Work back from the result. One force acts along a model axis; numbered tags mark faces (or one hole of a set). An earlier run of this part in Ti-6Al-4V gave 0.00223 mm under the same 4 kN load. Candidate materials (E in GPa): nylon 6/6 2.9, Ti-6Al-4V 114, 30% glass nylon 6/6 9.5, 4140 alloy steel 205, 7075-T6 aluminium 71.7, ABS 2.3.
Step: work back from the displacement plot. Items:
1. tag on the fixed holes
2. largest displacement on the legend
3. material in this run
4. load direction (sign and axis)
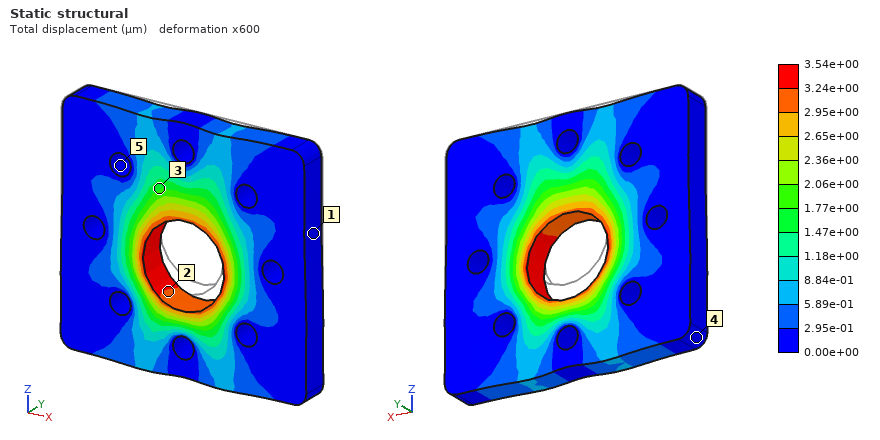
5
3.54e+00 µm
7075-T6 aluminium
-Z
